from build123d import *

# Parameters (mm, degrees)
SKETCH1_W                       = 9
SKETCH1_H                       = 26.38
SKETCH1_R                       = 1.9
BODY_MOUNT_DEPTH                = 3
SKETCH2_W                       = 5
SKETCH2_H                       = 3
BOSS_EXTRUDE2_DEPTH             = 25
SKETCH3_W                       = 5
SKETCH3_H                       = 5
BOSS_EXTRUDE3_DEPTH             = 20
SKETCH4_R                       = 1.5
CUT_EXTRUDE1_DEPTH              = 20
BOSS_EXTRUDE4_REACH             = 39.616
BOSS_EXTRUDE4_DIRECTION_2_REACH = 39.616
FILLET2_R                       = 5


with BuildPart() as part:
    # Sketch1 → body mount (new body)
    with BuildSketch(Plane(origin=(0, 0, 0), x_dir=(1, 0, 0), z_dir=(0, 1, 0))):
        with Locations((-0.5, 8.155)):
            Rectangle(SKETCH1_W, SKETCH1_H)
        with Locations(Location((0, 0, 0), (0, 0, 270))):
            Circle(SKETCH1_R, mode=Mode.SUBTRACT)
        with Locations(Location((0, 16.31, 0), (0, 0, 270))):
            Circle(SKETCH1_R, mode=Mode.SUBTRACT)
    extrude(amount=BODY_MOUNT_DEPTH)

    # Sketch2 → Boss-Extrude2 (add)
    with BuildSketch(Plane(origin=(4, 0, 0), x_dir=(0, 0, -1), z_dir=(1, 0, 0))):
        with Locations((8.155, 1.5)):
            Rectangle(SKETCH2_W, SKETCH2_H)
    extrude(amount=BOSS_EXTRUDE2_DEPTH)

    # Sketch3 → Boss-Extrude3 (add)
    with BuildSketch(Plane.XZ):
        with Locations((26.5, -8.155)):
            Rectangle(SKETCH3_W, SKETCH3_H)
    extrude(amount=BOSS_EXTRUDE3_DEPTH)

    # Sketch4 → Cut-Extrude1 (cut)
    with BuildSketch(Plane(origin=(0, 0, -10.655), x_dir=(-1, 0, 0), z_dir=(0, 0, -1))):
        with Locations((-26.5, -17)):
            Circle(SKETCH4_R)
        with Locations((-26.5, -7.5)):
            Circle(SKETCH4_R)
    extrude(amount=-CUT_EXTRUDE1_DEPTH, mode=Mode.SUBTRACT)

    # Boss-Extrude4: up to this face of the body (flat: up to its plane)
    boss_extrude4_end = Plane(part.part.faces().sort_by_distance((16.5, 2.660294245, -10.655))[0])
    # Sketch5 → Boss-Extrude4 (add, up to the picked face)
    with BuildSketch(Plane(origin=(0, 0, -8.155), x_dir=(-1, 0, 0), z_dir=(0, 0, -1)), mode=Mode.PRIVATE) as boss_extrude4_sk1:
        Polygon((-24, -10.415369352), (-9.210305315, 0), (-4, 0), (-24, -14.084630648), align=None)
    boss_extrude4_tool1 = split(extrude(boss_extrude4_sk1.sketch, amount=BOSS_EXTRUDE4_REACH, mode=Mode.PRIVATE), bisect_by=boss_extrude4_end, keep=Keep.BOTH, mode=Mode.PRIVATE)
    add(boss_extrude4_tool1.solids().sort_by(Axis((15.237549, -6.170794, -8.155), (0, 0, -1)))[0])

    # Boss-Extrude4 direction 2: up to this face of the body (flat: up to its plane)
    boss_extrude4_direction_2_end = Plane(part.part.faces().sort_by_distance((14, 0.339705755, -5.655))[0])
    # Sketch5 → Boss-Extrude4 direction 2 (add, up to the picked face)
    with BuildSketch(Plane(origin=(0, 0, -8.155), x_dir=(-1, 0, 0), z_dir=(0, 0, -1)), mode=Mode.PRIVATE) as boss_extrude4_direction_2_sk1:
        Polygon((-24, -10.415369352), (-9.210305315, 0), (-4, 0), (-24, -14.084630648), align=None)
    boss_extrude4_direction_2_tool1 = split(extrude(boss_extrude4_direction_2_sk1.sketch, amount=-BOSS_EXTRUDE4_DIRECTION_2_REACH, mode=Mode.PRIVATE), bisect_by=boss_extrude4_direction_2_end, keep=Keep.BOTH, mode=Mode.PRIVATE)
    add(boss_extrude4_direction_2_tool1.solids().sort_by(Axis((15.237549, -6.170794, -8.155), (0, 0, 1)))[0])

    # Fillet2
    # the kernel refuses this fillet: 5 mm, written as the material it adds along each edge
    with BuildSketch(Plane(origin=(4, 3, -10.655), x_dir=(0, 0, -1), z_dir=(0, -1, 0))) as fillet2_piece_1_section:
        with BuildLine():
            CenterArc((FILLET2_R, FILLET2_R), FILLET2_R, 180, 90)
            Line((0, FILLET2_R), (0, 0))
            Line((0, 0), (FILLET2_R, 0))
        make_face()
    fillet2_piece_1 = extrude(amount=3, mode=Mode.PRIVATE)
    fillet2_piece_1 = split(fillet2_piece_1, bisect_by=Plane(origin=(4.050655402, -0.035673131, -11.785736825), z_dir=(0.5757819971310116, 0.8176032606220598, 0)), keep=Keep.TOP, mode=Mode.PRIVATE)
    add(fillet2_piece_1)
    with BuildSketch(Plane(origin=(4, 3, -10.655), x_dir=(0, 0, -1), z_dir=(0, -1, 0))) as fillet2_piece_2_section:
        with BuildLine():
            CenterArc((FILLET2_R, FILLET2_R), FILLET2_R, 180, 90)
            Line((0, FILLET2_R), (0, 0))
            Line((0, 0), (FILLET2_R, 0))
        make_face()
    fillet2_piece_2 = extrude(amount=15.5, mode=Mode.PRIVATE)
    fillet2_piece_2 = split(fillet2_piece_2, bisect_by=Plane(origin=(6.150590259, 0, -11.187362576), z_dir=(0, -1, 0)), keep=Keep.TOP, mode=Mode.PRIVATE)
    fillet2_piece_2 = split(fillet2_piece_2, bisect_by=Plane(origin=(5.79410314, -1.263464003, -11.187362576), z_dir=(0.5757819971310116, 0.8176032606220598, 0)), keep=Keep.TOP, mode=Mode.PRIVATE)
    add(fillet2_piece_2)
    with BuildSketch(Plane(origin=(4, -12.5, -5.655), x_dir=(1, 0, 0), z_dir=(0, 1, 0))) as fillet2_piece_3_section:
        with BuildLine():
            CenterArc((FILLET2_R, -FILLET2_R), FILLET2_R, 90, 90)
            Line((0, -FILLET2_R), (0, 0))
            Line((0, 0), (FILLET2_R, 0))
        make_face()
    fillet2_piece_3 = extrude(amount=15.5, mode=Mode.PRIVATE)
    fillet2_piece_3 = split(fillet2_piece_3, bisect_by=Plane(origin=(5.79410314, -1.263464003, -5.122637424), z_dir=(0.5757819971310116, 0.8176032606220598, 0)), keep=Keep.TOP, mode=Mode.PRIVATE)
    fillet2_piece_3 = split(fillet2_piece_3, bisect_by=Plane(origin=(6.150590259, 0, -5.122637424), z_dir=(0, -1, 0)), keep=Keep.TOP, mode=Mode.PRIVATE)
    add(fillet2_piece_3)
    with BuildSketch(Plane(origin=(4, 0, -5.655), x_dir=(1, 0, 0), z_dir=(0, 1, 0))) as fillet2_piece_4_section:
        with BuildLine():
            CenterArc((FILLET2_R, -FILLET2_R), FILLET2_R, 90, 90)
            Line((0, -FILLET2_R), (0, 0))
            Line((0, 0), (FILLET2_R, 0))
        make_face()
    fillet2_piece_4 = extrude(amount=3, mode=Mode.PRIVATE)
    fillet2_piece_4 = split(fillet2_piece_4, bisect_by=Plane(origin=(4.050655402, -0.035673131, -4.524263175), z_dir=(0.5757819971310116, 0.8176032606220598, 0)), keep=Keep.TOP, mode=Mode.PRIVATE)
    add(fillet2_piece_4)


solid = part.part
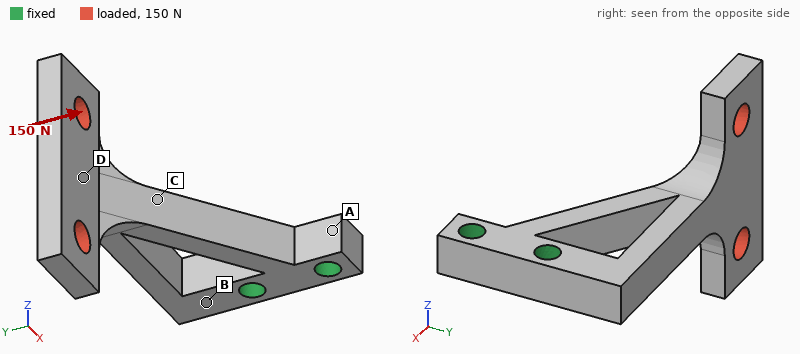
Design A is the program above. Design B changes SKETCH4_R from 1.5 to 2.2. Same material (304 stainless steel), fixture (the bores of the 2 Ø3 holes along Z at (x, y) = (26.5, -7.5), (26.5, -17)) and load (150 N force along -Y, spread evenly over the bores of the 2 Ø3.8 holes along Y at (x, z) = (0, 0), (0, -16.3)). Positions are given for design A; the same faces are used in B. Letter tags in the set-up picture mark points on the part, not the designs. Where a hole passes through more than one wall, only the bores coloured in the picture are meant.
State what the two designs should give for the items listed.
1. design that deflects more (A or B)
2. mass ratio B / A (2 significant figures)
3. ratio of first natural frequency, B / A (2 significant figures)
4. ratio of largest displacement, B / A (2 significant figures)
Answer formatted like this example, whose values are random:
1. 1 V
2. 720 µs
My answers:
1. A
2. 0.96
3. 1.0
4. 0.89
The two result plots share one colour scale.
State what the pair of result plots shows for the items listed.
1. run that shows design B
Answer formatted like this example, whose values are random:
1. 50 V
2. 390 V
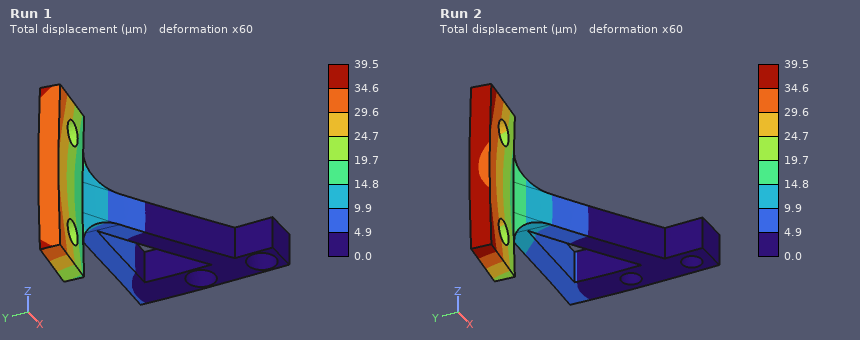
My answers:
1. Run 1
